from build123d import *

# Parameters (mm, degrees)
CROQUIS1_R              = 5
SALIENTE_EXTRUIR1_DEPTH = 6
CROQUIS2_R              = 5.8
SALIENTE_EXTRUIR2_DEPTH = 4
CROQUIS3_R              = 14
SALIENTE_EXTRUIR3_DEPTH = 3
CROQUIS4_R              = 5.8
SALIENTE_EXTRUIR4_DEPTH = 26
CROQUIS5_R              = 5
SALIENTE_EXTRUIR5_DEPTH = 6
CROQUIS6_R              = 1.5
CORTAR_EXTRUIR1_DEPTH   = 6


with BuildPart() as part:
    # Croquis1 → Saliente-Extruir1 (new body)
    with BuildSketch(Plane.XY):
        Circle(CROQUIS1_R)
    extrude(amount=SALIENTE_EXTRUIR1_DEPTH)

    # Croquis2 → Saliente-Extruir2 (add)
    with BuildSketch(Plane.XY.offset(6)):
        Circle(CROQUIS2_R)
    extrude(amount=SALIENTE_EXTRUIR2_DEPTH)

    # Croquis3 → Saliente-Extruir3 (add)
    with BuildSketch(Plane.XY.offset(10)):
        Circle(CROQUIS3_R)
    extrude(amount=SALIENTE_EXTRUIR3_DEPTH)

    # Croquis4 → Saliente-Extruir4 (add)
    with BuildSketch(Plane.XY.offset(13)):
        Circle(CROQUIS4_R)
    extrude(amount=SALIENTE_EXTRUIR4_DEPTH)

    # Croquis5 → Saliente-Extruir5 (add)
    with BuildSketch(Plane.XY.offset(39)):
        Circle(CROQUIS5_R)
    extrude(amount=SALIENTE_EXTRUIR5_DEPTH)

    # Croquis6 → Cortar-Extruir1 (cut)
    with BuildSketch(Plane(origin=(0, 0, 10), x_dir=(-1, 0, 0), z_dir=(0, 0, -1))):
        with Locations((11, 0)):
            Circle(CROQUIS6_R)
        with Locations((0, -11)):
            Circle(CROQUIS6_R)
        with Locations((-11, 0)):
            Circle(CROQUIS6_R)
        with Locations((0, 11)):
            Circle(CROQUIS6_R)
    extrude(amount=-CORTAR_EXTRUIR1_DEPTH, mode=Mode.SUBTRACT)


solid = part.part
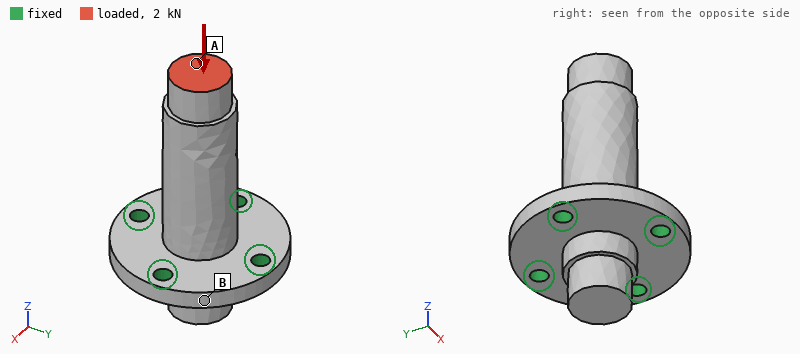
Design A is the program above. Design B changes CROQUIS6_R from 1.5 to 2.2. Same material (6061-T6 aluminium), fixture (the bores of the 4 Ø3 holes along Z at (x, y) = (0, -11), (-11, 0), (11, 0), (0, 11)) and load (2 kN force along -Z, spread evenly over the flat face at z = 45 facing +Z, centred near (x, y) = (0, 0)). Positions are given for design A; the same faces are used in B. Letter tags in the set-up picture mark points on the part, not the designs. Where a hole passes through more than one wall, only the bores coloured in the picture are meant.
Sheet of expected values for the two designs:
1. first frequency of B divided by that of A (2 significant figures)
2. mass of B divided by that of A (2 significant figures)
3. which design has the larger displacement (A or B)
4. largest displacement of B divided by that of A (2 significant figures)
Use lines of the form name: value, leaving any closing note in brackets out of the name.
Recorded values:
first frequency of B divided by that of A: 1.1
mass of B divided by that of A: 0.98
which design has the larger displacement: A
largest displacement of B divided by that of A: 0.87
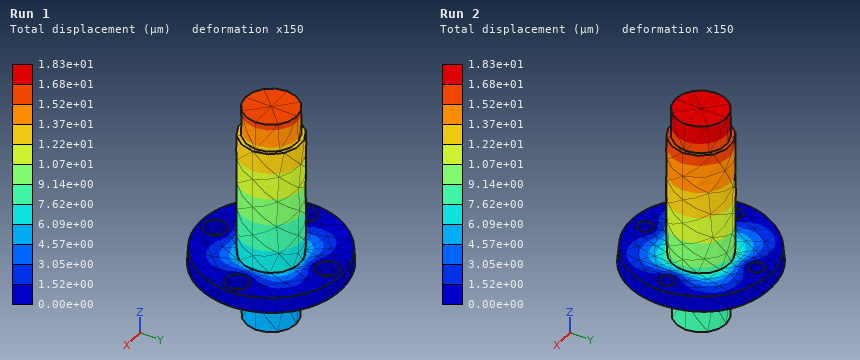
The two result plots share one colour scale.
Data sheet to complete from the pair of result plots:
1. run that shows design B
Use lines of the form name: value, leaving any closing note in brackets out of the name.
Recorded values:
run that shows design B: Run 1
